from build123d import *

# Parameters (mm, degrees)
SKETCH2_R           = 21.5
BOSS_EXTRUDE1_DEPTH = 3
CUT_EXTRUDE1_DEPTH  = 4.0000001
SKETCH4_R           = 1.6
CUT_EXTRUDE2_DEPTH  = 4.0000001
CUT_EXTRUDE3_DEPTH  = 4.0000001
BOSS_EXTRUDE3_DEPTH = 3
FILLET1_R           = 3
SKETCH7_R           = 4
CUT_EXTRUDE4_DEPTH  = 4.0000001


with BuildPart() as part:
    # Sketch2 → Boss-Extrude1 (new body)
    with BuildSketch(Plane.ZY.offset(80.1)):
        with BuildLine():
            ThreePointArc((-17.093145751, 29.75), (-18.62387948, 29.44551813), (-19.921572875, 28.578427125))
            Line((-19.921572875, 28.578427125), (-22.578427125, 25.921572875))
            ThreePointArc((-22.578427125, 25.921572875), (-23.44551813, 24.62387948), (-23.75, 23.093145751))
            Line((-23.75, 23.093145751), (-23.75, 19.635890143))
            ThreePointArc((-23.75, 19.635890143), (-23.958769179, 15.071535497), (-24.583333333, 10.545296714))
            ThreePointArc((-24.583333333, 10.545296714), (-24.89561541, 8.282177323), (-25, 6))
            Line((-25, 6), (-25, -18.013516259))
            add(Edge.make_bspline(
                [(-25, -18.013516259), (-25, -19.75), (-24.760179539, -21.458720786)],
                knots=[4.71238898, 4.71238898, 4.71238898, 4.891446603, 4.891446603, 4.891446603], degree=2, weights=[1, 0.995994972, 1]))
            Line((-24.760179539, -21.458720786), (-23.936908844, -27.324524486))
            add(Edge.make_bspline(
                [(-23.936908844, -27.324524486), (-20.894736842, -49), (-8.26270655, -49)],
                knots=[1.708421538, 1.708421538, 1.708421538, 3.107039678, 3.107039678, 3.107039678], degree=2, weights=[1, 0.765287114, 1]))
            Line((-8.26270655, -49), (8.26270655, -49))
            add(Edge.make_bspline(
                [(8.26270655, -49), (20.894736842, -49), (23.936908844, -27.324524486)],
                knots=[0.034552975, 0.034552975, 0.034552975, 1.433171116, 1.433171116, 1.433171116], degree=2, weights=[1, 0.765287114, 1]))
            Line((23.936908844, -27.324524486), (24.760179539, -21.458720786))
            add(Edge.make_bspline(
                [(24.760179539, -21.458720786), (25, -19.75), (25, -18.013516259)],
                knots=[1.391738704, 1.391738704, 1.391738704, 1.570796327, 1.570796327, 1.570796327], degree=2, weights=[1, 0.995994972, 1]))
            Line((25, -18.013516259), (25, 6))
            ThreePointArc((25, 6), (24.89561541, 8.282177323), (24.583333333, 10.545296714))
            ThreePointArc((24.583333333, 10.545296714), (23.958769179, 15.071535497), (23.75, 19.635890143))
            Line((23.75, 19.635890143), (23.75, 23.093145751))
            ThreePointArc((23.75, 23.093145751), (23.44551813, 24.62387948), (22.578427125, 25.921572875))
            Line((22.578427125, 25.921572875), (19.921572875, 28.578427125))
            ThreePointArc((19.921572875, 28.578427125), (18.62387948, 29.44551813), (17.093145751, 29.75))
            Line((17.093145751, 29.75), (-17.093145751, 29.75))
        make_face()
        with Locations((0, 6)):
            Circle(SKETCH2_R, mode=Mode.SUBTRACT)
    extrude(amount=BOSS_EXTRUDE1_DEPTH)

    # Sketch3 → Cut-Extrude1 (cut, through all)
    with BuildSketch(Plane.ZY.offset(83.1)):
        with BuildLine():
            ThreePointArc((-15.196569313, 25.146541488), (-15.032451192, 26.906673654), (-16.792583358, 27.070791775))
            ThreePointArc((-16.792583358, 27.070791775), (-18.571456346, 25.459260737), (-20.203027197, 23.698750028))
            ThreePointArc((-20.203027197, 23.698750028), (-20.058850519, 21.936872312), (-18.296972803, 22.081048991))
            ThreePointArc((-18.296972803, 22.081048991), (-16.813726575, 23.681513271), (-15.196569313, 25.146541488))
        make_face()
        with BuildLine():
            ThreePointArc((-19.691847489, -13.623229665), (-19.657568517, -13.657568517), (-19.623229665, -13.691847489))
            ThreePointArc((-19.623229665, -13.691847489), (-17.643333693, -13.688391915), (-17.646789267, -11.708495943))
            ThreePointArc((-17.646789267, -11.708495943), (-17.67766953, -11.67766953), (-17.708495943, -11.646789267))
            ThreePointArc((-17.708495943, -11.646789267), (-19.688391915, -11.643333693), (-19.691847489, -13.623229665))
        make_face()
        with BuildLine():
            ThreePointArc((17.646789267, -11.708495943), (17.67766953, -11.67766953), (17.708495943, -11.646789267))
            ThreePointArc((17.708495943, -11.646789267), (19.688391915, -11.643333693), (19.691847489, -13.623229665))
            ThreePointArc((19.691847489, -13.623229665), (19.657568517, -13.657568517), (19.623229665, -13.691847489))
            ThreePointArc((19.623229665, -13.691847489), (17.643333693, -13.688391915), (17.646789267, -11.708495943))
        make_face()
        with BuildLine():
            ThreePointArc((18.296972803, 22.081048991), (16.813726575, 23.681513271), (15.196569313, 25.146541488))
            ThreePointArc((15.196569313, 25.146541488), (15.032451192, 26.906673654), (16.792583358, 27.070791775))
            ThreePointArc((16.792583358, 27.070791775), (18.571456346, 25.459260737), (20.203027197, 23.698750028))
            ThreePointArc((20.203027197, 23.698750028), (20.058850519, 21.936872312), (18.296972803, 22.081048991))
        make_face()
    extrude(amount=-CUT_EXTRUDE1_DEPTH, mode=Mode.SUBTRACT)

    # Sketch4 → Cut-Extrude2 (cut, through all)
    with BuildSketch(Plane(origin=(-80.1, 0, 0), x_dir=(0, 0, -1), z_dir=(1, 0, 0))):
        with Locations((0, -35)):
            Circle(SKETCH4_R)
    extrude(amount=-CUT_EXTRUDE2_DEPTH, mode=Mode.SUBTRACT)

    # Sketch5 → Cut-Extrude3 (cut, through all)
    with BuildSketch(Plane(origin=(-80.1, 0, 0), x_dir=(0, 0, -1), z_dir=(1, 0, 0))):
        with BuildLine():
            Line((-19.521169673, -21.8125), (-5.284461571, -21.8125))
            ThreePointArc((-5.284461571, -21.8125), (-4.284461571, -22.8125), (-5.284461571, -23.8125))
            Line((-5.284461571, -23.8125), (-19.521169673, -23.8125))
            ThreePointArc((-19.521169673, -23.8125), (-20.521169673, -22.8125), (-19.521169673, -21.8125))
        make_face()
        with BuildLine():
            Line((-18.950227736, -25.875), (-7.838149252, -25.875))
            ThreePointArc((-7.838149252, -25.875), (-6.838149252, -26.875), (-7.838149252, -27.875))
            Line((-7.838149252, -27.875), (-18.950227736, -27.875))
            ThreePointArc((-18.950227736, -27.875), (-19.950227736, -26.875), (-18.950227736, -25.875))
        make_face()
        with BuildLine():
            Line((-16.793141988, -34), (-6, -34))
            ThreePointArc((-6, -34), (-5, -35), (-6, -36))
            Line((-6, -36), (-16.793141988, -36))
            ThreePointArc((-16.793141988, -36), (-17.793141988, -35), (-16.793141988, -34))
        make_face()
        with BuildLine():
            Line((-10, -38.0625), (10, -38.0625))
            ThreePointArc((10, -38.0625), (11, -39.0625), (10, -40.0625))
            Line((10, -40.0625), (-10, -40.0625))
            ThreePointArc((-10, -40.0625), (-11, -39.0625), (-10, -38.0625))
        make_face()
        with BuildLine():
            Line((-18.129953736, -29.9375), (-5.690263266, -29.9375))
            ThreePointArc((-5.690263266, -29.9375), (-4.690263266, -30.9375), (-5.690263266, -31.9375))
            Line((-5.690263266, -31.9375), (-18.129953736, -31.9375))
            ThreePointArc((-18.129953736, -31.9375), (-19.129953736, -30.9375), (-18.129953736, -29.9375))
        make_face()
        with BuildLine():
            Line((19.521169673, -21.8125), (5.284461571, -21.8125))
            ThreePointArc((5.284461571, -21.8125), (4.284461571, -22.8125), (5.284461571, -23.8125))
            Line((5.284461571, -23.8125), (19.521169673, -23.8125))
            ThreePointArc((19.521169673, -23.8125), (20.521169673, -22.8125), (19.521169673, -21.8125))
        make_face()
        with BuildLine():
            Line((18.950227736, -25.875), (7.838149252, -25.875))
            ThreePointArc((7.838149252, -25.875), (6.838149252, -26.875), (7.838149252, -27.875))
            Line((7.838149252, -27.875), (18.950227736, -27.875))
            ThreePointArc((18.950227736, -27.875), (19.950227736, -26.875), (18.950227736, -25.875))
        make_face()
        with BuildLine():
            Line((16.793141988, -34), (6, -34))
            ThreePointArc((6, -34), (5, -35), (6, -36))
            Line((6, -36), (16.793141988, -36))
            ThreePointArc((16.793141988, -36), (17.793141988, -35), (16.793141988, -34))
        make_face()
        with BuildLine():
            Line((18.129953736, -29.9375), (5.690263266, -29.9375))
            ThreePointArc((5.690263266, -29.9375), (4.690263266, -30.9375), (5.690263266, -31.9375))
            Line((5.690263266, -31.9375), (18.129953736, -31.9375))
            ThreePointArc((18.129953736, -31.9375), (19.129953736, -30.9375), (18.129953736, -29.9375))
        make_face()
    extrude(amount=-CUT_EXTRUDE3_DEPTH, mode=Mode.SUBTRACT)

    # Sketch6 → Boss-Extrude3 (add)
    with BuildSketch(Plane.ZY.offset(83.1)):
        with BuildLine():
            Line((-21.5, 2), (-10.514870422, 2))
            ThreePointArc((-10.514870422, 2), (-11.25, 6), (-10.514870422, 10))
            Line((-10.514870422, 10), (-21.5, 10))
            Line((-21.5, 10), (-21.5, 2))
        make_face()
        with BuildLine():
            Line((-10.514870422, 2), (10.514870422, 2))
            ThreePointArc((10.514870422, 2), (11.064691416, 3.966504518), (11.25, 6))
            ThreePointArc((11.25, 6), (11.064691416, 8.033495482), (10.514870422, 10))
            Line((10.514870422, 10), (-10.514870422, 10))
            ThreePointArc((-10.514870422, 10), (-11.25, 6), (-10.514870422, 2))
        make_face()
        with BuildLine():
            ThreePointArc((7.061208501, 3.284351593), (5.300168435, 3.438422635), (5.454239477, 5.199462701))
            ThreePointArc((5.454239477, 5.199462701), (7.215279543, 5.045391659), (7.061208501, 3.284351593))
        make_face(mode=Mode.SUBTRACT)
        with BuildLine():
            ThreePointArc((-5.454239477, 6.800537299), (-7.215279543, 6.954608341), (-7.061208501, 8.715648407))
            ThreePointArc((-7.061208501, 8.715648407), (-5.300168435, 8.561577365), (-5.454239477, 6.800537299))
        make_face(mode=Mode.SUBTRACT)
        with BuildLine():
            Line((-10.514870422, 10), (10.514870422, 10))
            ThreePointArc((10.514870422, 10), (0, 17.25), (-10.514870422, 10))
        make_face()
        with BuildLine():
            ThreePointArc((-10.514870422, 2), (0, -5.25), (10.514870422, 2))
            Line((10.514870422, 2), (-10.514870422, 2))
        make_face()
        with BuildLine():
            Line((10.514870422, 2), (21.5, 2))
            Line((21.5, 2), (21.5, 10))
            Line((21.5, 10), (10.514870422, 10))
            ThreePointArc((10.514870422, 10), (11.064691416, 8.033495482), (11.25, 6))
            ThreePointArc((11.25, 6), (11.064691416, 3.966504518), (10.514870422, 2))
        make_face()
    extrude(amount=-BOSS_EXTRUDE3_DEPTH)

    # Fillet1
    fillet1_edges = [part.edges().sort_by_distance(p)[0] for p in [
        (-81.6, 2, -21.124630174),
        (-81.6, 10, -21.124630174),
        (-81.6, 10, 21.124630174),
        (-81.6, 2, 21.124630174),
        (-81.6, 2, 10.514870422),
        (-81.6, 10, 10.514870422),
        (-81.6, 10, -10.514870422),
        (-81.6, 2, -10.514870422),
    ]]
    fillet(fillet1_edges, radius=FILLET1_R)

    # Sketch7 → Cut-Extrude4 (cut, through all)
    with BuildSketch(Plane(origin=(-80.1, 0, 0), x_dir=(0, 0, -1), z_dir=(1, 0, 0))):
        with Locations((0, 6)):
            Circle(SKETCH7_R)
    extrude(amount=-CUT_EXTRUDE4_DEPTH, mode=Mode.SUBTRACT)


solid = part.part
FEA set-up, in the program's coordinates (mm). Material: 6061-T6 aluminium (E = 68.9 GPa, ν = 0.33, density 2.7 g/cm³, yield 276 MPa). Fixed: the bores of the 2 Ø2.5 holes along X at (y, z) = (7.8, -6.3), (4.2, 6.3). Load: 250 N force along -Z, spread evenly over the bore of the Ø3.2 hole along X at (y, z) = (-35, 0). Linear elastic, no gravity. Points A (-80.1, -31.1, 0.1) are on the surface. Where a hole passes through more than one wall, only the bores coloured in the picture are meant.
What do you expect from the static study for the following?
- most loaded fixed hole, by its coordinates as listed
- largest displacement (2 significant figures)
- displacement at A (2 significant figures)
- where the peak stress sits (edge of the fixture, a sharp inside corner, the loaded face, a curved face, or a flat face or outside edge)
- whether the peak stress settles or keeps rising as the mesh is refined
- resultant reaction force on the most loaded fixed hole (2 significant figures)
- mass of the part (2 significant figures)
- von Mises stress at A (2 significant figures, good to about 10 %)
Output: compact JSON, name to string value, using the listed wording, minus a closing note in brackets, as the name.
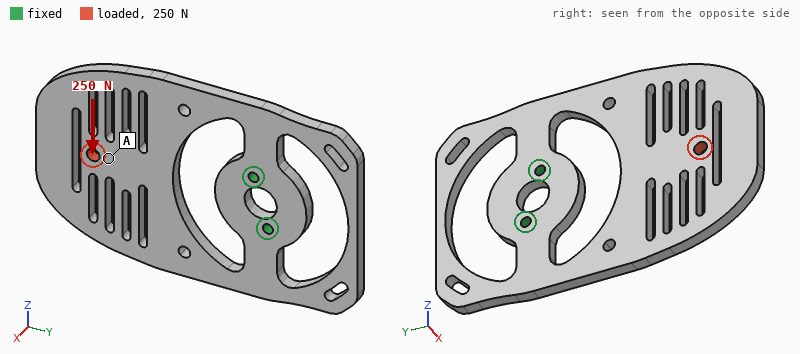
{"most loaded fixed hole, by its coordinates as listed": "(4.2, 6.3)", "largest displacement": "0.15 mm", "displacement at A": "0.11 mm", "where the peak stress sits": "edge of the fixture", "whether the peak stress settles or keeps rising as the mesh is refined": "keeps rising", "resultant reaction force on the most loaded fixed hole": "670 N", "mass of the part": "19 g", "von Mises stress at A": "11 MPa"}
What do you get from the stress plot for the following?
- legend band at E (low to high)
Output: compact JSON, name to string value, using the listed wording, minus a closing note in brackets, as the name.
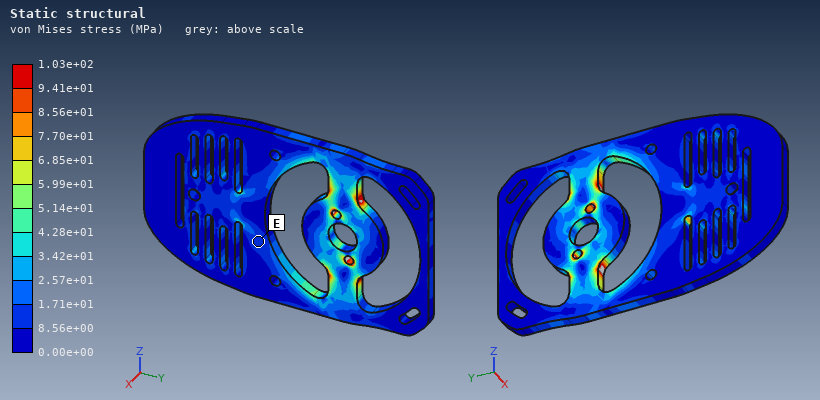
{"legend band at E": "8.56e+00 to 1.71e+01 MPa"}
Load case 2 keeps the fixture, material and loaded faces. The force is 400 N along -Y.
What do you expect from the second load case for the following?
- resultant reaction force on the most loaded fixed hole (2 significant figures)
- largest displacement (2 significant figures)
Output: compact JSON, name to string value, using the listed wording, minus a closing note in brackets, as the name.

{"resultant reaction force on the most loaded fixed hole": "210 N", "largest displacement": "41 µm"}
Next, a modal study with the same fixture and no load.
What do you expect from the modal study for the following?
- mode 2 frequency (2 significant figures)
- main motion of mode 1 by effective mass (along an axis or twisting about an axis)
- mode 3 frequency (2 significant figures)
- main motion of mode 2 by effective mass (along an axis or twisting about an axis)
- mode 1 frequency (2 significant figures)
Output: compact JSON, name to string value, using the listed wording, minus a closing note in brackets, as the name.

{"mode 2 frequency": "1600 Hz", "main motion of mode 1 by effective mass": "along X", "mode 3 frequency": "2000 Hz", "main motion of mode 2 by effective mass": "twisting about Y", "mode 1 frequency": "410 Hz"}
